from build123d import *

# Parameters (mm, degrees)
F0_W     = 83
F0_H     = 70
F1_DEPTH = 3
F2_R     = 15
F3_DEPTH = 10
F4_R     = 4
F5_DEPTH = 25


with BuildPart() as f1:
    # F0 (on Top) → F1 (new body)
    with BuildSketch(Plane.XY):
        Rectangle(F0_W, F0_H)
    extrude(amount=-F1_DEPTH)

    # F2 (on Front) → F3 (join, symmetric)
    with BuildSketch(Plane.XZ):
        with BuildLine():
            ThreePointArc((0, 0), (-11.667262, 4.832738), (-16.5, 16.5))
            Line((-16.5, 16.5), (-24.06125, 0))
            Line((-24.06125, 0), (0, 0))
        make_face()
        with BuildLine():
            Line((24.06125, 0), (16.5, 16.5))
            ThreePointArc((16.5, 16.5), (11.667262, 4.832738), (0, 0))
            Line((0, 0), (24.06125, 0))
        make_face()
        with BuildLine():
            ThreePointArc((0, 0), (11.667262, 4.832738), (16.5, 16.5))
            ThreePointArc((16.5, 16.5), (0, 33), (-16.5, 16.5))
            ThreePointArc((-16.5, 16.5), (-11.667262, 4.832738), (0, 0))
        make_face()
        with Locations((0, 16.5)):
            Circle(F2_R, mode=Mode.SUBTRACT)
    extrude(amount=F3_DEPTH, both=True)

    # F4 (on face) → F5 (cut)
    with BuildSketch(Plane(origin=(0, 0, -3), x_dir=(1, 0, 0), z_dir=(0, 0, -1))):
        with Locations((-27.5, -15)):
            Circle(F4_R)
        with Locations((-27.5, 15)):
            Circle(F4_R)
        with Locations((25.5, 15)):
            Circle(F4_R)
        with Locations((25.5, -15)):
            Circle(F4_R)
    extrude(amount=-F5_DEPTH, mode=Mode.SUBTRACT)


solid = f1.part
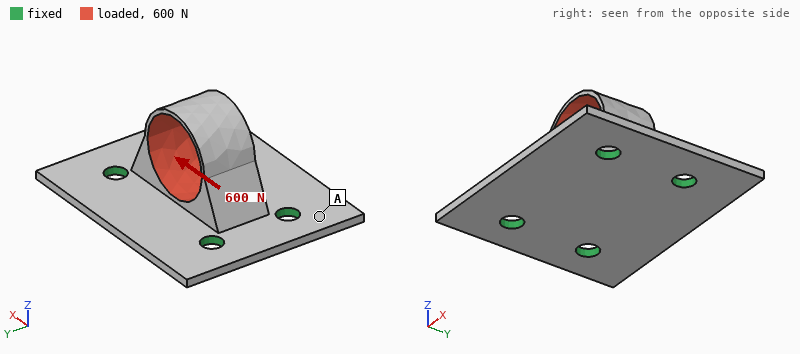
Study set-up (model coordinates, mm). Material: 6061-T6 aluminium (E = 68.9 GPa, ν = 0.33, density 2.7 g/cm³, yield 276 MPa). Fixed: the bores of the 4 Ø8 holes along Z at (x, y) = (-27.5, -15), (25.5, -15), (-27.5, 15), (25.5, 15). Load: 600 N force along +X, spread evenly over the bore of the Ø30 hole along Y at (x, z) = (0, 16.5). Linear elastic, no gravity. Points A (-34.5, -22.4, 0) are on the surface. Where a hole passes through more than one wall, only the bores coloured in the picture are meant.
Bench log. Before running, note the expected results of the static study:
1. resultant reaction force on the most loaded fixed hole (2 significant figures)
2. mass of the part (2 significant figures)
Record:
200 N
66 g
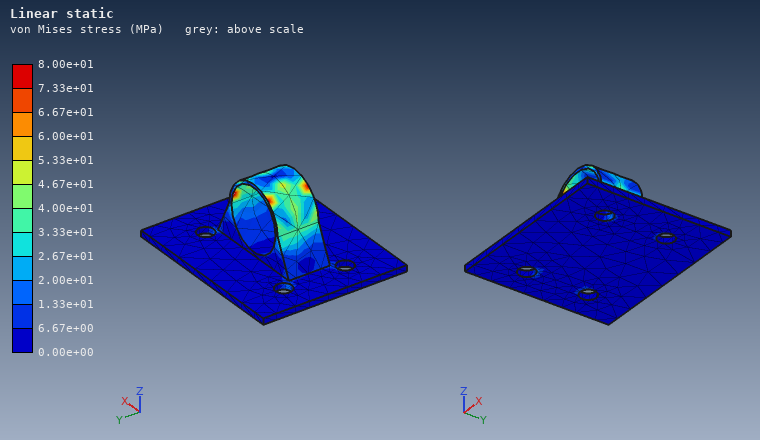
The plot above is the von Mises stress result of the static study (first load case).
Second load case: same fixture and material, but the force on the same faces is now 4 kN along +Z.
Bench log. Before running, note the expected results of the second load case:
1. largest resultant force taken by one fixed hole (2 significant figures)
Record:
1.2 kN
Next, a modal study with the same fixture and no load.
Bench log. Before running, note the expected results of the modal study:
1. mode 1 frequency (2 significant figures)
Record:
5400 Hz
